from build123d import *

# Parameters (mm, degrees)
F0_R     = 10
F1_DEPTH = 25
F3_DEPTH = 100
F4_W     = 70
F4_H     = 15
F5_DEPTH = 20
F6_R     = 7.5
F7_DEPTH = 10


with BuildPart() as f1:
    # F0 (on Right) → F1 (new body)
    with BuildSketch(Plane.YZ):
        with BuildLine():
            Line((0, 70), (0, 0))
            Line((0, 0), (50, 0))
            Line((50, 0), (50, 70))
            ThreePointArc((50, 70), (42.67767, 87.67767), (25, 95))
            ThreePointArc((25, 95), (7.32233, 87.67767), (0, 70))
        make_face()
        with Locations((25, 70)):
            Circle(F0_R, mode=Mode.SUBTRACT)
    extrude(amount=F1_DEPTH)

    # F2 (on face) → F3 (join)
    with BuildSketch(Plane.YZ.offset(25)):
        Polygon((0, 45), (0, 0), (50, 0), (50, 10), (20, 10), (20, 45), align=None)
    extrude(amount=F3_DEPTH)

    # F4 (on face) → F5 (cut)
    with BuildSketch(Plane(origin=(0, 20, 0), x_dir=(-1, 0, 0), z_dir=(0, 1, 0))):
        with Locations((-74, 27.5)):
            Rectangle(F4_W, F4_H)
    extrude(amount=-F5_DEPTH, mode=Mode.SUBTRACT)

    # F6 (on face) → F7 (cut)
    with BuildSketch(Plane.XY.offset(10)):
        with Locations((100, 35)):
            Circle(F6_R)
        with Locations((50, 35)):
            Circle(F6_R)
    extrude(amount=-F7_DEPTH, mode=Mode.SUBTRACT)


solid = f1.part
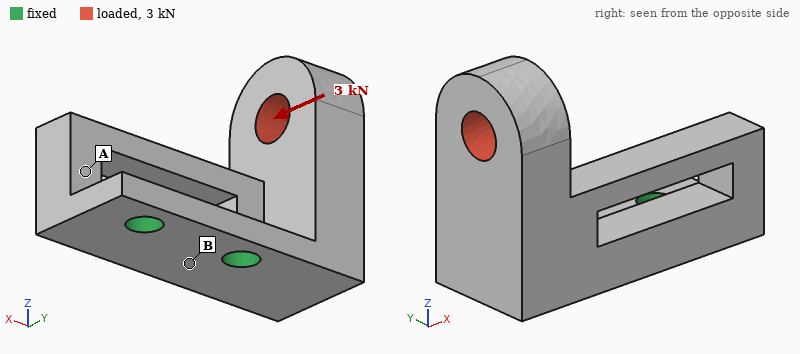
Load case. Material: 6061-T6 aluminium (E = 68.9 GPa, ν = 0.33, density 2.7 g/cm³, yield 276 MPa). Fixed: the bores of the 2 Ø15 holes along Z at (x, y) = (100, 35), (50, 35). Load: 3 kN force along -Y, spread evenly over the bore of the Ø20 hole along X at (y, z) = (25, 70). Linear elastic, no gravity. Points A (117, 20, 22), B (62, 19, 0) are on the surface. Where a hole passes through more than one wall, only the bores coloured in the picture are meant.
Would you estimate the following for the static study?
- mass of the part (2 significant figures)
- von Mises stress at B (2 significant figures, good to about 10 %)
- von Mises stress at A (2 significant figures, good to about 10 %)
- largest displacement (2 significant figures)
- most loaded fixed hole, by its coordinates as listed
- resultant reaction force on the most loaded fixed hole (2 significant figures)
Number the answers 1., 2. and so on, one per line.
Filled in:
1. 540 g
2. 60 MPa
3. 28 MPa
4. 0.55 mm
5. (50, 35)
6. 4.1 kN
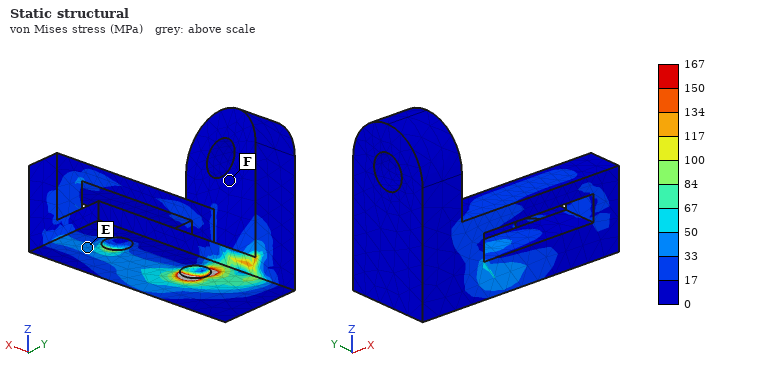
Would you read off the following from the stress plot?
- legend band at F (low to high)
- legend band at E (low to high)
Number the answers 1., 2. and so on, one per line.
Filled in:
1. 0 to 17 MPa
2. 33 to 50 MPa
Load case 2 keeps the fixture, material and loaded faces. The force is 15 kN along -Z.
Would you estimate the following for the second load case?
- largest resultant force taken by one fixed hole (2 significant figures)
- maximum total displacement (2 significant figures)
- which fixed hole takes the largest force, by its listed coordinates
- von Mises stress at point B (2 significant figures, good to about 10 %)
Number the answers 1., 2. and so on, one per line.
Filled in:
1. 20 kN
2. 0.75 mm
3. (50, 35)
4. 74 MPa
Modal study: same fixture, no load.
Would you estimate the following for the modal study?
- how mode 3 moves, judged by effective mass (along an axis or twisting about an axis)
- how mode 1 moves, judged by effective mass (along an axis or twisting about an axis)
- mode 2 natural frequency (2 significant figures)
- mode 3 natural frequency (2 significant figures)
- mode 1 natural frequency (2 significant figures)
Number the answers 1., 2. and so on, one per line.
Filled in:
1. along Z
2. along Y
3. 1500 Hz
4. 3400 Hz
5. 1000 Hz
